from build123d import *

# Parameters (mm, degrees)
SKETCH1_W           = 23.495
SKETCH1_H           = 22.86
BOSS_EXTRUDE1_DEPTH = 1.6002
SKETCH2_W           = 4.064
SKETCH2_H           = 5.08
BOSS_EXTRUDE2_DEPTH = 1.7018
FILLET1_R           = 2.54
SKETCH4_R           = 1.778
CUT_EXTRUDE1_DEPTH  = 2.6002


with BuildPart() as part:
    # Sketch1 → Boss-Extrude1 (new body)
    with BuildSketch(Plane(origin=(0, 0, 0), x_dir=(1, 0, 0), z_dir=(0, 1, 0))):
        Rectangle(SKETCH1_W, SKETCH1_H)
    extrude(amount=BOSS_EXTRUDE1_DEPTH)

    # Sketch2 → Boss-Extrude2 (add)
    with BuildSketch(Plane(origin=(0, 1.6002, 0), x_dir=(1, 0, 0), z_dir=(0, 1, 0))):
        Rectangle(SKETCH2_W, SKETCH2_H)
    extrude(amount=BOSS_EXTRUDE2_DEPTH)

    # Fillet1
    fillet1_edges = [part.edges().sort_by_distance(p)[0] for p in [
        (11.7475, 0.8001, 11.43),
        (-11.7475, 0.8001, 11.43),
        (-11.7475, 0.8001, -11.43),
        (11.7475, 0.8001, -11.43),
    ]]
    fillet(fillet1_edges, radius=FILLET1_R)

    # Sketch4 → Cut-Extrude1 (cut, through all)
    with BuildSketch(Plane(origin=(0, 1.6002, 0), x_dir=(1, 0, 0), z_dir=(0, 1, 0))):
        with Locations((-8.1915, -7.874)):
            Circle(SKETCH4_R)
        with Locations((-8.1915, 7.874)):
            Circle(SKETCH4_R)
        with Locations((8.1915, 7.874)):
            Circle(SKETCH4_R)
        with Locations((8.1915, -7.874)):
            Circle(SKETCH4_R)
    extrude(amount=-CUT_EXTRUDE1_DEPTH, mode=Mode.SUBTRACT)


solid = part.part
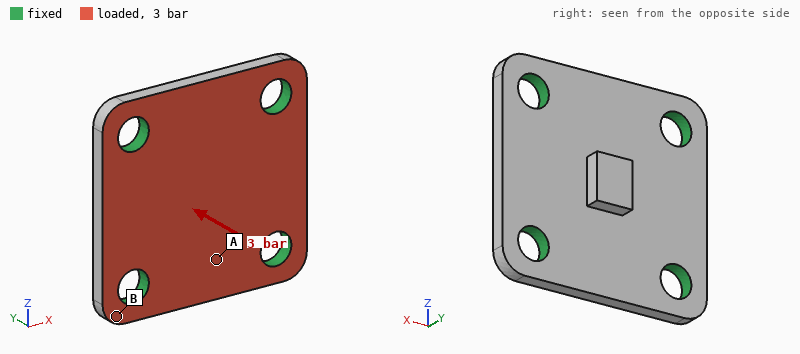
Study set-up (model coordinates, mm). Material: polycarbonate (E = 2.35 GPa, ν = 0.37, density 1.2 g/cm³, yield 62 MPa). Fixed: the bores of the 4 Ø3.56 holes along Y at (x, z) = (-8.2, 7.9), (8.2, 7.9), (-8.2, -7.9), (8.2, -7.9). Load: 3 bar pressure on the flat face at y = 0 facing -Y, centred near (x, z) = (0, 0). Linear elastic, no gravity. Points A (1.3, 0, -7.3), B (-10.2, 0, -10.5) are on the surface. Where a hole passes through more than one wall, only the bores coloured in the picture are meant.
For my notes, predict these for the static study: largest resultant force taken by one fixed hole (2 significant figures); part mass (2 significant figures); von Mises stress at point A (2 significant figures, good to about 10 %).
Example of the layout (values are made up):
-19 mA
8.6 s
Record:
37 N
0.99 g
5.5 MPa
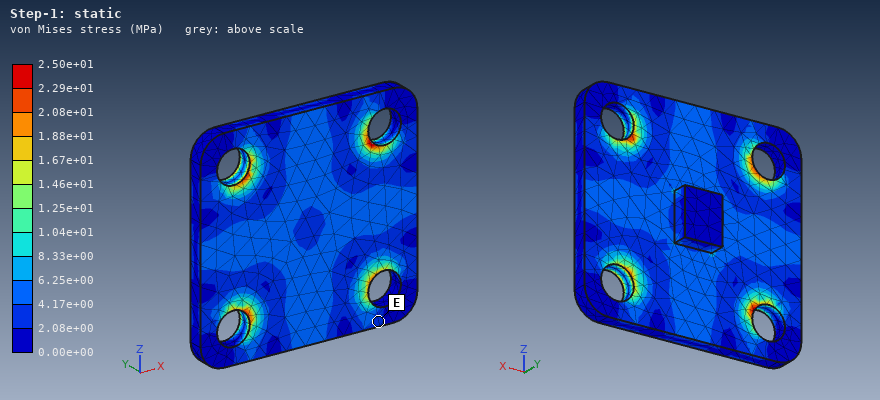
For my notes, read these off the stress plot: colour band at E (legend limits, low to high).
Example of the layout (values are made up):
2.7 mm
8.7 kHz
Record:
2.08e+00 to 4.17e+00 MPa
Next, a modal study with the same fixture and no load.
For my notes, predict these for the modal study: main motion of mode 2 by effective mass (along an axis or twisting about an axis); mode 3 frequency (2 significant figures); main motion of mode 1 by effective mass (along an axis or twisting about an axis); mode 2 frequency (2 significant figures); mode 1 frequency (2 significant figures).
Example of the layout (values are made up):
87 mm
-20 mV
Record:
twisting about X
12 kHz
along Y
12 kHz
7900 Hz
